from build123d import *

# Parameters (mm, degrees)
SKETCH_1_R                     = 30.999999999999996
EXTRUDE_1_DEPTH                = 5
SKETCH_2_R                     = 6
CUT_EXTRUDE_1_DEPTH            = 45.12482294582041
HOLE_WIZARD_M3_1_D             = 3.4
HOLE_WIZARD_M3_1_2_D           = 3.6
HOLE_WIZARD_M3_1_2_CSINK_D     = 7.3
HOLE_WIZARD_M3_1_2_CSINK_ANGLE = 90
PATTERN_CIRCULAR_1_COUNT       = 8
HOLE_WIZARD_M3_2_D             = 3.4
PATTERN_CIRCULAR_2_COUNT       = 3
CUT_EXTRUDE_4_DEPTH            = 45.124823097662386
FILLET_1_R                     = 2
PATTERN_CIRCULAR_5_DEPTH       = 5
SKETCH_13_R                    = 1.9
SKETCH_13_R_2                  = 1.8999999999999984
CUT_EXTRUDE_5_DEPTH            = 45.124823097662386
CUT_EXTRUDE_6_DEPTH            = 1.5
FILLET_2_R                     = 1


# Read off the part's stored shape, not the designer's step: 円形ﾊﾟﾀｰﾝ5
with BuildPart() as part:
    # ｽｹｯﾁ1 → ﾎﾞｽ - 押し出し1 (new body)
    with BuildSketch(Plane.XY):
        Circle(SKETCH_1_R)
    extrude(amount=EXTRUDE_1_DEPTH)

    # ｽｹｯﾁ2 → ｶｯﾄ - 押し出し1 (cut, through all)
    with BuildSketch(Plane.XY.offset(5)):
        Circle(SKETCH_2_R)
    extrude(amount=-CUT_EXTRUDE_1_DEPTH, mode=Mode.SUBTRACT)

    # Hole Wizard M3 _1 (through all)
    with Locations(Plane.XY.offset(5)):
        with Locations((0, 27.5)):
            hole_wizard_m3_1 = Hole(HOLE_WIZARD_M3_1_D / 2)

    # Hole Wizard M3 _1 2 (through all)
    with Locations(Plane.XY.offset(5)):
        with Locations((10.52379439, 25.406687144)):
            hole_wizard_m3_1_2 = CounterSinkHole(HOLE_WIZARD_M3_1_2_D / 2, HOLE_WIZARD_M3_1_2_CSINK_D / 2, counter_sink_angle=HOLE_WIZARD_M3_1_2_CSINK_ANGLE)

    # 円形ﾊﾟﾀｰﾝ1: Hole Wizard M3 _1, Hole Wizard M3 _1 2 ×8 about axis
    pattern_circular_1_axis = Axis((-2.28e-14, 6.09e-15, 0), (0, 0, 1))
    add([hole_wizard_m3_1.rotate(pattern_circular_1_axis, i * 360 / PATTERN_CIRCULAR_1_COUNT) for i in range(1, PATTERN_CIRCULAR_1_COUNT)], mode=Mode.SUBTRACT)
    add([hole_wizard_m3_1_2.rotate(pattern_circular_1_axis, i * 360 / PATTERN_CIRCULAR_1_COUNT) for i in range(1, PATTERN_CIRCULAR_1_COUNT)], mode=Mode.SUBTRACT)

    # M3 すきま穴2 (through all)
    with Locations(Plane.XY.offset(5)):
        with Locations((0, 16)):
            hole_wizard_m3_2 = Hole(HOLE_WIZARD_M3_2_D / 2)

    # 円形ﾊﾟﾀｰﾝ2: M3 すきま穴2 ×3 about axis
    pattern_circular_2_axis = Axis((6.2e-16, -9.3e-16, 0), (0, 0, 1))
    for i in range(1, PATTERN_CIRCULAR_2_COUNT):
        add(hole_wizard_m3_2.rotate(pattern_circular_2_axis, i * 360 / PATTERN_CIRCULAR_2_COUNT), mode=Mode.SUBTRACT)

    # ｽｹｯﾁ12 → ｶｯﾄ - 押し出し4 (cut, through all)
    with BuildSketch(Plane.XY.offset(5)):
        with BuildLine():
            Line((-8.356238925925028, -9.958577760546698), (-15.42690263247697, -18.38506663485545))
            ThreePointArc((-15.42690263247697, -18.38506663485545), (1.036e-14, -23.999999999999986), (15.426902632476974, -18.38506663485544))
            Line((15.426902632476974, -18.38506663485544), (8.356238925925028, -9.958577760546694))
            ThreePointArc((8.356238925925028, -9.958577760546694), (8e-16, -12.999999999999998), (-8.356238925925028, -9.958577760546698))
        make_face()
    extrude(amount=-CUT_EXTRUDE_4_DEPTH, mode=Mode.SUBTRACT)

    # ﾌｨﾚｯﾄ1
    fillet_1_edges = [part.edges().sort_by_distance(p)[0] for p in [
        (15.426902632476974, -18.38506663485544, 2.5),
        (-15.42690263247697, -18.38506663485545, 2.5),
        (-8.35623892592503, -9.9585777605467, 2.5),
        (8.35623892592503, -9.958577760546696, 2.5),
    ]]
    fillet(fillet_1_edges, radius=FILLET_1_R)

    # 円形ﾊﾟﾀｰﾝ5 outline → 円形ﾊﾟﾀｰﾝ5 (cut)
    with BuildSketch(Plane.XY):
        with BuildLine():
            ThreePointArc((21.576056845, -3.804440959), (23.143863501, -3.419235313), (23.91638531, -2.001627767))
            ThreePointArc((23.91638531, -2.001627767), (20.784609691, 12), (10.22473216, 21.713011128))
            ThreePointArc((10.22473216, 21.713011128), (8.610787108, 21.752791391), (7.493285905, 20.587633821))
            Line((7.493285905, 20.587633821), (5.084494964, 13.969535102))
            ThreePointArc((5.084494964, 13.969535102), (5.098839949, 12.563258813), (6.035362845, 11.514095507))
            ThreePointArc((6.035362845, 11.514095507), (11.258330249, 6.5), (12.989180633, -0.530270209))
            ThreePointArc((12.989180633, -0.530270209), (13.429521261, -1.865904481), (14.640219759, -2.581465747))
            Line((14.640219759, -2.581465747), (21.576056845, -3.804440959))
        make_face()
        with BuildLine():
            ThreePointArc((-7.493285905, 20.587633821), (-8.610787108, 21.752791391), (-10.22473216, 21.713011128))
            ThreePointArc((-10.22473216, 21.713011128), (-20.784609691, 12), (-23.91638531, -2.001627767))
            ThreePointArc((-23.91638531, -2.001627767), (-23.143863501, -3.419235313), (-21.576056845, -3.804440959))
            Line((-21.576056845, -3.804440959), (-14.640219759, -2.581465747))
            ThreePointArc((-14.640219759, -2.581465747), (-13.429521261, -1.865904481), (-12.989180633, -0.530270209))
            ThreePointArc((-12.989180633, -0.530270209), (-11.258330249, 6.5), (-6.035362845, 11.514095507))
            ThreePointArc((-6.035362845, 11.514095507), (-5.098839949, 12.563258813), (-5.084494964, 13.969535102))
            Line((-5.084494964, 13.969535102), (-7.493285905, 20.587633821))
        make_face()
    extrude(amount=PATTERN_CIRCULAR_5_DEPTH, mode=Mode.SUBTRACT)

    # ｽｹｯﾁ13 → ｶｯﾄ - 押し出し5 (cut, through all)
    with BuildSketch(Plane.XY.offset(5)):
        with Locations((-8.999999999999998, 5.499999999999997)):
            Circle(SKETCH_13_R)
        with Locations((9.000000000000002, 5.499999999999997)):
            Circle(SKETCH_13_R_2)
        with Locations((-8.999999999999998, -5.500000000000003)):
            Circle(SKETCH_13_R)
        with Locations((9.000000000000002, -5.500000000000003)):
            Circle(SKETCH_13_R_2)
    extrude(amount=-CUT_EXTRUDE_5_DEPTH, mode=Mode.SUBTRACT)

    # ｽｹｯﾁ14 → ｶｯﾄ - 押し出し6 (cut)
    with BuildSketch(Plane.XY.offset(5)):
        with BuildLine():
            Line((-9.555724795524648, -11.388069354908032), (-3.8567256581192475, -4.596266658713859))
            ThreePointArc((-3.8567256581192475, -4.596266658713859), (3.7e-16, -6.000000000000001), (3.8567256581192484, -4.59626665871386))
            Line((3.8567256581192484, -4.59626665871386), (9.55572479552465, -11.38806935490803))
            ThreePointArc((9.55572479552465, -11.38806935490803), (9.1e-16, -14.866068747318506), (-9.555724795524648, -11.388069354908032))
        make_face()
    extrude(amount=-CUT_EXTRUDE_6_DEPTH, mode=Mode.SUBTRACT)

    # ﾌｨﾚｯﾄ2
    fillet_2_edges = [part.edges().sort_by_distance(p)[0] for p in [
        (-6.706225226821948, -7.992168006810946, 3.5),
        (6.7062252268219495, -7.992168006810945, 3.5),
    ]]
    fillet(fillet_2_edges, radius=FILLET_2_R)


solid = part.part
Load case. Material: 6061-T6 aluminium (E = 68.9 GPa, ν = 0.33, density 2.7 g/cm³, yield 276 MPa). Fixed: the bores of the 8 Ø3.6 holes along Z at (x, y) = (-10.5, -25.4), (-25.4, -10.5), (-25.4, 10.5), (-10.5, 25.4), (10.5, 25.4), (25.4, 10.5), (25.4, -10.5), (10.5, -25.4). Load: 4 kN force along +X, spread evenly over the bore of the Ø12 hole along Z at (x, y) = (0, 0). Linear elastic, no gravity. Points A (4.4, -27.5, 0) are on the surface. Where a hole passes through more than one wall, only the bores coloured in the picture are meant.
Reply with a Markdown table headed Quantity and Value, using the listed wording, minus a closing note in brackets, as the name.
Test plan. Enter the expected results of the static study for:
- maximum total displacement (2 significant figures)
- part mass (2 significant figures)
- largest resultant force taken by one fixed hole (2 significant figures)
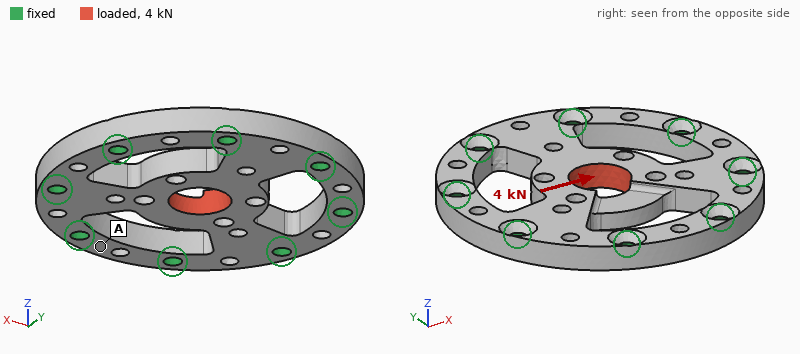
| Quantity | Value |
|---|---|
| maximum total displacement | 29 µm |
| part mass | 24 g |
| largest resultant force taken by one fixed hole | 1.5 kN |
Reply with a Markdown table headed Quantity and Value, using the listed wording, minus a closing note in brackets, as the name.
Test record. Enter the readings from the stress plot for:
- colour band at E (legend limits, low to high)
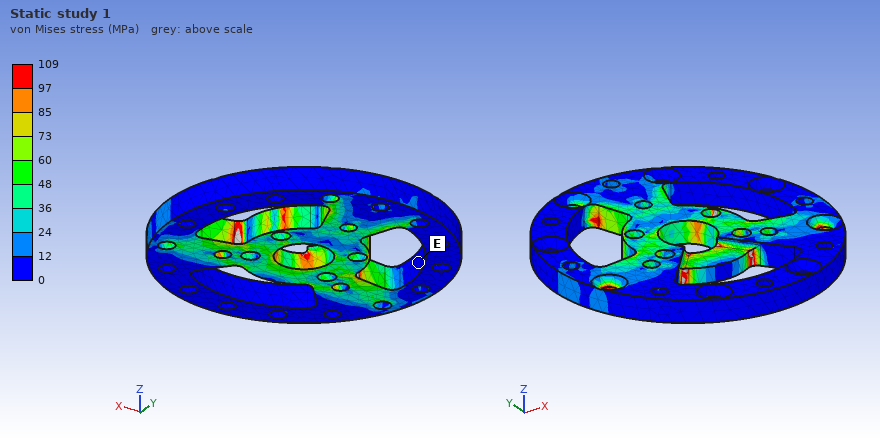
| Quantity | Value |
|---|---|
| colour band at E | 0 to 12 MPa |
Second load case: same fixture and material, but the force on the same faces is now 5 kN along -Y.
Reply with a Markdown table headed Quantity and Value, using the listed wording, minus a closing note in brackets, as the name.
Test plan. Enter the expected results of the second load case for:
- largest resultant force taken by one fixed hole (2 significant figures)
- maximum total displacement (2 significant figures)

| Quantity | Value |
|---|---|
| largest resultant force taken by one fixed hole | 1.4 kN |
| maximum total displacement | 45 µm |
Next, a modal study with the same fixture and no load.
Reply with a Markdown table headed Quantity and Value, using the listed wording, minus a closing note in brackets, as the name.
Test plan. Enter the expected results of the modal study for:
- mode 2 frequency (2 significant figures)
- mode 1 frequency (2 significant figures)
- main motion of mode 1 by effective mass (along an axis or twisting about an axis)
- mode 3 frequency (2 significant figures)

| Quantity | Value |
|---|---|
| mode 2 frequency | 17 kHz |
| mode 1 frequency | 9000 Hz |
| main motion of mode 1 by effective mass | along Z |
| mode 3 frequency | 17 kHz |
